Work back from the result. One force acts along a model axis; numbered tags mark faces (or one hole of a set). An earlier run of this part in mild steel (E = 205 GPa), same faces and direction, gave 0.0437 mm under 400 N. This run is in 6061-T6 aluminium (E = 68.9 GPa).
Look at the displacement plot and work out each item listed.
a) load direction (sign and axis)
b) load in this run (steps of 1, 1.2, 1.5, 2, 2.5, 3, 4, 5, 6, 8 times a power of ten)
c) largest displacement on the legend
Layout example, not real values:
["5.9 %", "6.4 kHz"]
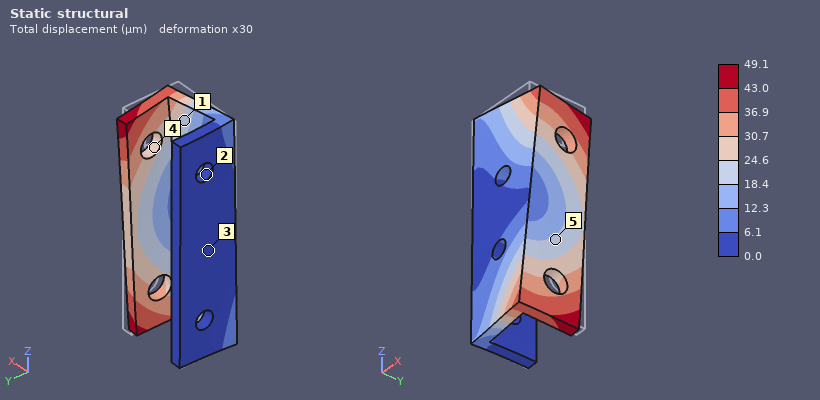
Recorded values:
["-Z", "150 N", "49.1 µm"]
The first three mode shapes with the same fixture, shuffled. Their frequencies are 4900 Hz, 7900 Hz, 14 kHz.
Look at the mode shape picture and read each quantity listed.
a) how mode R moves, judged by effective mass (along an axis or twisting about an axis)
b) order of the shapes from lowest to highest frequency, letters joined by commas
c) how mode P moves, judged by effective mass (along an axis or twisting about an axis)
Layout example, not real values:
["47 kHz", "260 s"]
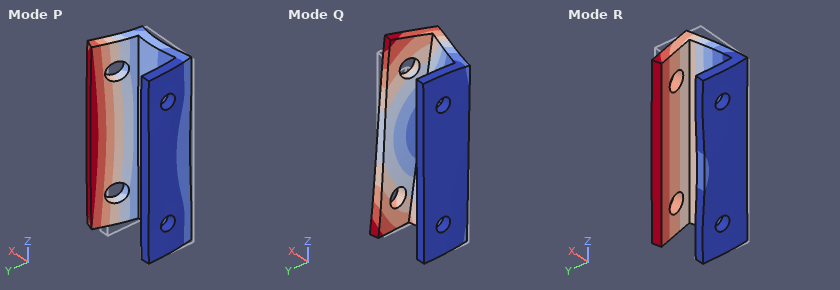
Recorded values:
["along Y", "R, Q, P", "along X"]
